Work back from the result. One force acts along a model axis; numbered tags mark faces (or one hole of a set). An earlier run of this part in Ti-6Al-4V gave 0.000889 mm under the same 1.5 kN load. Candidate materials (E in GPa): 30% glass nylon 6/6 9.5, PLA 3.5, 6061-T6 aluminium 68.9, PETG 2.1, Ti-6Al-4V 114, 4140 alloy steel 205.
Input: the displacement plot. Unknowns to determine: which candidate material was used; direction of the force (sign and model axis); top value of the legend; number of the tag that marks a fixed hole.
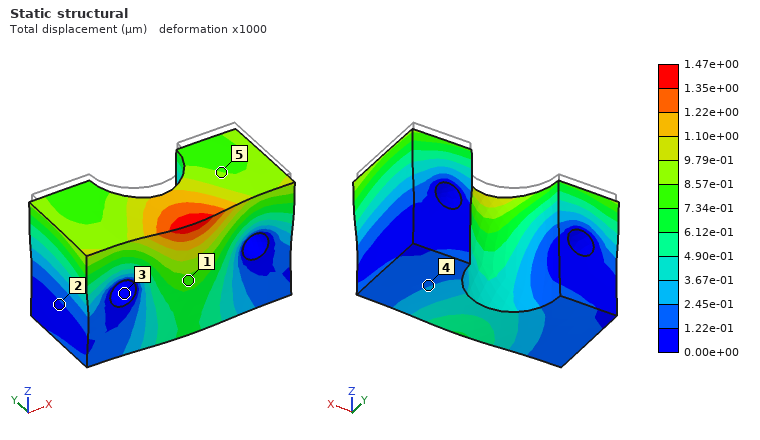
6061-T6 aluminium
-Z
1.47e+00 µm
3
